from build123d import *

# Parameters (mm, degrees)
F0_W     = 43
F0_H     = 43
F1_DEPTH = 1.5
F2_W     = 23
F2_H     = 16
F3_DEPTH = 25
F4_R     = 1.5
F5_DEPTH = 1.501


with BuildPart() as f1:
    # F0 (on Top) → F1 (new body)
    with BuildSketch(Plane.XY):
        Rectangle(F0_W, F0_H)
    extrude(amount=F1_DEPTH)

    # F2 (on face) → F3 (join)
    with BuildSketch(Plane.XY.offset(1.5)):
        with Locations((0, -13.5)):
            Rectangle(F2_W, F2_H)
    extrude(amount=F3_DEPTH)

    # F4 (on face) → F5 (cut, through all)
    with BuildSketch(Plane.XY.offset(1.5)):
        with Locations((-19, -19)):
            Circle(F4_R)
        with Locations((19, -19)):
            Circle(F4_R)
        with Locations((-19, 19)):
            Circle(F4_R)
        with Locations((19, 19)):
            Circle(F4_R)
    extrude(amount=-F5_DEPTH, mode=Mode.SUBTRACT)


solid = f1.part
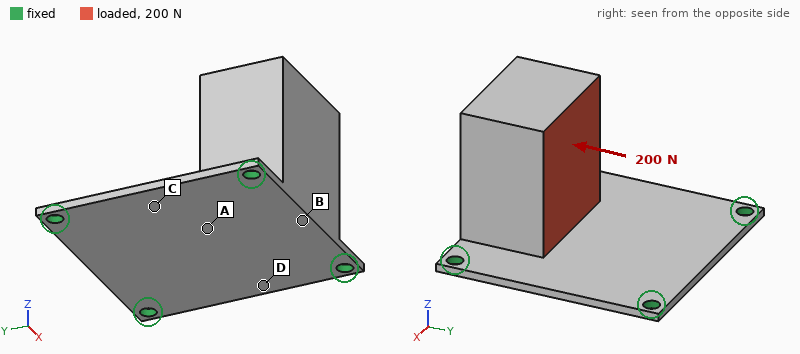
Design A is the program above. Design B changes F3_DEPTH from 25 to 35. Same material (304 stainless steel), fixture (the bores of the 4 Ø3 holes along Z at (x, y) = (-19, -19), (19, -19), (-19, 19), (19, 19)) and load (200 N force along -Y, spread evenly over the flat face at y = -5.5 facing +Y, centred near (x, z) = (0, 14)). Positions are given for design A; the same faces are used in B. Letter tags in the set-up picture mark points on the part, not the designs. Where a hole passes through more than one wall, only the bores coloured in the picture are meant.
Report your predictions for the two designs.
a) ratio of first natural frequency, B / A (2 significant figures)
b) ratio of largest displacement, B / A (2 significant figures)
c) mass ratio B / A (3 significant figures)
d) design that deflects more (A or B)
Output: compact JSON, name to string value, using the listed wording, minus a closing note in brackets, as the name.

{"ratio of first natural frequency, B / A": "0.64", "ratio of largest displacement, B / A": "1.8", "mass ratio B / A": "1.31", "design that deflects more": "B"}
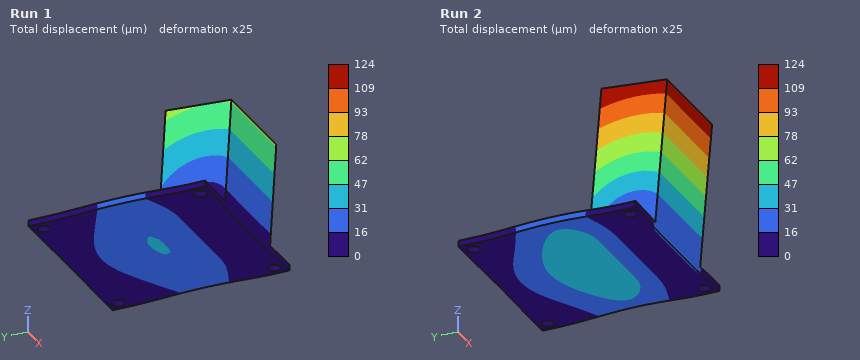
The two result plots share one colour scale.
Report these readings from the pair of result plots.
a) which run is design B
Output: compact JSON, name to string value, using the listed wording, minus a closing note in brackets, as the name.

{"which run is design B": "Run 2"}
